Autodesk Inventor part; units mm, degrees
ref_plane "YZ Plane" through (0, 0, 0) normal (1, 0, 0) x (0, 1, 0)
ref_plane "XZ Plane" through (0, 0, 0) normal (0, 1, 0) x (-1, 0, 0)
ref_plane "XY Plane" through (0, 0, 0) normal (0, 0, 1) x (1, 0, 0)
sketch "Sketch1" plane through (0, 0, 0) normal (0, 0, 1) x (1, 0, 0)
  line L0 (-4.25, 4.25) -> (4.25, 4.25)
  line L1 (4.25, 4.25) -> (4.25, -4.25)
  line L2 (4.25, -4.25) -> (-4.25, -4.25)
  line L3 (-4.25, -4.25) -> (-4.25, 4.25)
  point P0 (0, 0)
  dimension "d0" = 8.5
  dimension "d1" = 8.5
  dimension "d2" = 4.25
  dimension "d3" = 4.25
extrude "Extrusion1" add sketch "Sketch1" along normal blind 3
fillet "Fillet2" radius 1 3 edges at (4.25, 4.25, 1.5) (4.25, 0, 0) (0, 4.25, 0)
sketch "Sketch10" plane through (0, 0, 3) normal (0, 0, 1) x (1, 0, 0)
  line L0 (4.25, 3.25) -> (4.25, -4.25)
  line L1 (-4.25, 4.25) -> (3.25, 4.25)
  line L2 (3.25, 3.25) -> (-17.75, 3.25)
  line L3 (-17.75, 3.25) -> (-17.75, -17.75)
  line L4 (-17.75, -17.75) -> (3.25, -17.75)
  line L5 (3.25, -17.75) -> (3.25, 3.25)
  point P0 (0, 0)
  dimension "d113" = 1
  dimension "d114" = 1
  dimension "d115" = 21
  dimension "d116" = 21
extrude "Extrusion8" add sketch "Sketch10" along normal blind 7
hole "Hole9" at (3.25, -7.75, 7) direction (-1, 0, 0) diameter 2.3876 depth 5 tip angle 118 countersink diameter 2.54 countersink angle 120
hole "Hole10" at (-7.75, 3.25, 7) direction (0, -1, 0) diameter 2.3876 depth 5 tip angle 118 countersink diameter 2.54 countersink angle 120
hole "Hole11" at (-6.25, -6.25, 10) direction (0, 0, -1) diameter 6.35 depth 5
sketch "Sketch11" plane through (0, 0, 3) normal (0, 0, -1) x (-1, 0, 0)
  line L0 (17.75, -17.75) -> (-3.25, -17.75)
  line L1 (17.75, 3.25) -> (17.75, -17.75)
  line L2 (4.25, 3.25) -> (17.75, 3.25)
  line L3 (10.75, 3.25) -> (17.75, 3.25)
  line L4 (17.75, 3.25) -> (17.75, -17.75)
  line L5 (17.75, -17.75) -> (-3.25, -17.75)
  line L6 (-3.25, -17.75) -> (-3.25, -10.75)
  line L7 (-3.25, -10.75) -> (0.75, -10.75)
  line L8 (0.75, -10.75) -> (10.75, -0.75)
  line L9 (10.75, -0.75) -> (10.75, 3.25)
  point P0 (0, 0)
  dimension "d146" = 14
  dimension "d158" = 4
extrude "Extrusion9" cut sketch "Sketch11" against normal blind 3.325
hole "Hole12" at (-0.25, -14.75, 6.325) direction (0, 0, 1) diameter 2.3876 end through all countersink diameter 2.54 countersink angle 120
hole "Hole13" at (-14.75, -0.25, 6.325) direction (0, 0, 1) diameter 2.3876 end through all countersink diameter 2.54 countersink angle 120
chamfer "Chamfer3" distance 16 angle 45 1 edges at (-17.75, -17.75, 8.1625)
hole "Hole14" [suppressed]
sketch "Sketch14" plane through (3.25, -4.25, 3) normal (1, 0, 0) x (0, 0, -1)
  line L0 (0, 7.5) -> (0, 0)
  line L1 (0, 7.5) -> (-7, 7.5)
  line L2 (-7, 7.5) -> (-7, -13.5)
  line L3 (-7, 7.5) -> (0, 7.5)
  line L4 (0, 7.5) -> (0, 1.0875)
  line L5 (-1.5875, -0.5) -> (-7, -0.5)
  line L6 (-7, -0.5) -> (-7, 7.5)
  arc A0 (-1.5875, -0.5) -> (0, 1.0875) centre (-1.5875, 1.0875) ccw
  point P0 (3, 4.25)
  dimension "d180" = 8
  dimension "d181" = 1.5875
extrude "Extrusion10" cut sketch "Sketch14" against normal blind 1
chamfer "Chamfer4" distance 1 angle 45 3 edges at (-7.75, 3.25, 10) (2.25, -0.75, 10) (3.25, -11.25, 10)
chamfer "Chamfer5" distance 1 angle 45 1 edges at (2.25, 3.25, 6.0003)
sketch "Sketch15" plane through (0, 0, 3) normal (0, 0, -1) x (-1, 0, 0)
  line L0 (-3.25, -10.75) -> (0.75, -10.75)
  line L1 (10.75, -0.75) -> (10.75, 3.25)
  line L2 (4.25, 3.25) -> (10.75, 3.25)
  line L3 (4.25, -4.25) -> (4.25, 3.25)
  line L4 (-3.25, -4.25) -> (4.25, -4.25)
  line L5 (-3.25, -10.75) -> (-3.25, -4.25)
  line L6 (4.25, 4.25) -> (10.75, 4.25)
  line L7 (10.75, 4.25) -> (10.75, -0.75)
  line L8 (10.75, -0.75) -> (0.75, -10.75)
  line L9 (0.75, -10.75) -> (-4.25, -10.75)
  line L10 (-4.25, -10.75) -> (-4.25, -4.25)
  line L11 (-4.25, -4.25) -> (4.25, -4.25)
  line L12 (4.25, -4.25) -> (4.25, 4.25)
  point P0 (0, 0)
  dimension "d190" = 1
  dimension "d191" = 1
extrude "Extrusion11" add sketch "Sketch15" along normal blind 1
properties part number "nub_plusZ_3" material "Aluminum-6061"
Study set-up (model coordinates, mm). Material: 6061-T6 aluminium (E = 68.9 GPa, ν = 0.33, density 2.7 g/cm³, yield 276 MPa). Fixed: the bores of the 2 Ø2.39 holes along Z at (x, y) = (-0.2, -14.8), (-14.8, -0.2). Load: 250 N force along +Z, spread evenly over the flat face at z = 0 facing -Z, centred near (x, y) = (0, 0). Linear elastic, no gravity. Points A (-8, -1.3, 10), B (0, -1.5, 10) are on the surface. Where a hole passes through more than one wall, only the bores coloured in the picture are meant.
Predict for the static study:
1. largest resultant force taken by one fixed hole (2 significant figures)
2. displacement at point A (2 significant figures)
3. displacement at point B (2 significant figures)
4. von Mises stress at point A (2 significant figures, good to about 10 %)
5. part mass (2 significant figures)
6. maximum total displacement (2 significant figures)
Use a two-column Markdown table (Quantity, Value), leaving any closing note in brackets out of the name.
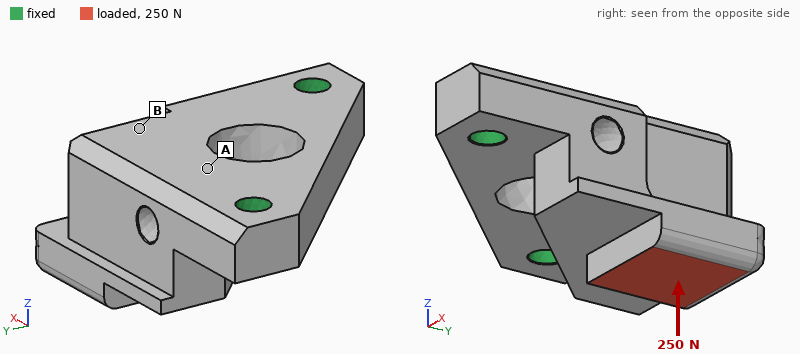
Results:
| Quantity | Value |
|---|---|
| largest resultant force taken by one fixed hole | 130 N |
| displacement at point A | 8.3 µm |
| displacement at point B | 24 µm |
| von Mises stress at point A | 33 MPa |
| part mass | 4.5 g |
| maximum total displacement | 47 µm |
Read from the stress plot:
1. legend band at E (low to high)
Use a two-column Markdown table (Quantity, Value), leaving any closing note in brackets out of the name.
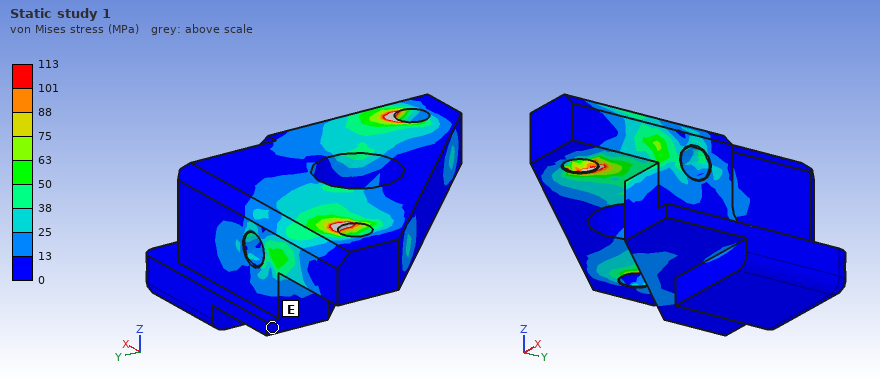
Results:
| Quantity | Value |
|---|---|
| legend band at E | 0 to 13 MPa |
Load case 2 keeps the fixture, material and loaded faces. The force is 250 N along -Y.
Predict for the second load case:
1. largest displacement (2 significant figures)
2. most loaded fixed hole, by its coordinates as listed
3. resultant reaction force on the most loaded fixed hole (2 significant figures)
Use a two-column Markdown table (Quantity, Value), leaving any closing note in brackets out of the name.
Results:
| Quantity | Value |
|---|---|
| largest displacement | 35 µm |
| most loaded fixed hole, by its coordinates as listed | (-0.2, -14.8) |
| resultant reaction force on the most loaded fixed hole | 220 N |
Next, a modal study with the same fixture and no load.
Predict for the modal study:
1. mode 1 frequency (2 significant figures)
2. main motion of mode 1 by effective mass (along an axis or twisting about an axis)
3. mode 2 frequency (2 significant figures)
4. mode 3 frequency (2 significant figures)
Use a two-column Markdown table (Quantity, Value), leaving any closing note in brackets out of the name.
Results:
| Quantity | Value |
|---|---|
| mode 1 frequency | 9900 Hz |
| main motion of mode 1 by effective mass | along Z |
| mode 2 frequency | 35 kHz |
| mode 3 frequency | 36 kHz |
